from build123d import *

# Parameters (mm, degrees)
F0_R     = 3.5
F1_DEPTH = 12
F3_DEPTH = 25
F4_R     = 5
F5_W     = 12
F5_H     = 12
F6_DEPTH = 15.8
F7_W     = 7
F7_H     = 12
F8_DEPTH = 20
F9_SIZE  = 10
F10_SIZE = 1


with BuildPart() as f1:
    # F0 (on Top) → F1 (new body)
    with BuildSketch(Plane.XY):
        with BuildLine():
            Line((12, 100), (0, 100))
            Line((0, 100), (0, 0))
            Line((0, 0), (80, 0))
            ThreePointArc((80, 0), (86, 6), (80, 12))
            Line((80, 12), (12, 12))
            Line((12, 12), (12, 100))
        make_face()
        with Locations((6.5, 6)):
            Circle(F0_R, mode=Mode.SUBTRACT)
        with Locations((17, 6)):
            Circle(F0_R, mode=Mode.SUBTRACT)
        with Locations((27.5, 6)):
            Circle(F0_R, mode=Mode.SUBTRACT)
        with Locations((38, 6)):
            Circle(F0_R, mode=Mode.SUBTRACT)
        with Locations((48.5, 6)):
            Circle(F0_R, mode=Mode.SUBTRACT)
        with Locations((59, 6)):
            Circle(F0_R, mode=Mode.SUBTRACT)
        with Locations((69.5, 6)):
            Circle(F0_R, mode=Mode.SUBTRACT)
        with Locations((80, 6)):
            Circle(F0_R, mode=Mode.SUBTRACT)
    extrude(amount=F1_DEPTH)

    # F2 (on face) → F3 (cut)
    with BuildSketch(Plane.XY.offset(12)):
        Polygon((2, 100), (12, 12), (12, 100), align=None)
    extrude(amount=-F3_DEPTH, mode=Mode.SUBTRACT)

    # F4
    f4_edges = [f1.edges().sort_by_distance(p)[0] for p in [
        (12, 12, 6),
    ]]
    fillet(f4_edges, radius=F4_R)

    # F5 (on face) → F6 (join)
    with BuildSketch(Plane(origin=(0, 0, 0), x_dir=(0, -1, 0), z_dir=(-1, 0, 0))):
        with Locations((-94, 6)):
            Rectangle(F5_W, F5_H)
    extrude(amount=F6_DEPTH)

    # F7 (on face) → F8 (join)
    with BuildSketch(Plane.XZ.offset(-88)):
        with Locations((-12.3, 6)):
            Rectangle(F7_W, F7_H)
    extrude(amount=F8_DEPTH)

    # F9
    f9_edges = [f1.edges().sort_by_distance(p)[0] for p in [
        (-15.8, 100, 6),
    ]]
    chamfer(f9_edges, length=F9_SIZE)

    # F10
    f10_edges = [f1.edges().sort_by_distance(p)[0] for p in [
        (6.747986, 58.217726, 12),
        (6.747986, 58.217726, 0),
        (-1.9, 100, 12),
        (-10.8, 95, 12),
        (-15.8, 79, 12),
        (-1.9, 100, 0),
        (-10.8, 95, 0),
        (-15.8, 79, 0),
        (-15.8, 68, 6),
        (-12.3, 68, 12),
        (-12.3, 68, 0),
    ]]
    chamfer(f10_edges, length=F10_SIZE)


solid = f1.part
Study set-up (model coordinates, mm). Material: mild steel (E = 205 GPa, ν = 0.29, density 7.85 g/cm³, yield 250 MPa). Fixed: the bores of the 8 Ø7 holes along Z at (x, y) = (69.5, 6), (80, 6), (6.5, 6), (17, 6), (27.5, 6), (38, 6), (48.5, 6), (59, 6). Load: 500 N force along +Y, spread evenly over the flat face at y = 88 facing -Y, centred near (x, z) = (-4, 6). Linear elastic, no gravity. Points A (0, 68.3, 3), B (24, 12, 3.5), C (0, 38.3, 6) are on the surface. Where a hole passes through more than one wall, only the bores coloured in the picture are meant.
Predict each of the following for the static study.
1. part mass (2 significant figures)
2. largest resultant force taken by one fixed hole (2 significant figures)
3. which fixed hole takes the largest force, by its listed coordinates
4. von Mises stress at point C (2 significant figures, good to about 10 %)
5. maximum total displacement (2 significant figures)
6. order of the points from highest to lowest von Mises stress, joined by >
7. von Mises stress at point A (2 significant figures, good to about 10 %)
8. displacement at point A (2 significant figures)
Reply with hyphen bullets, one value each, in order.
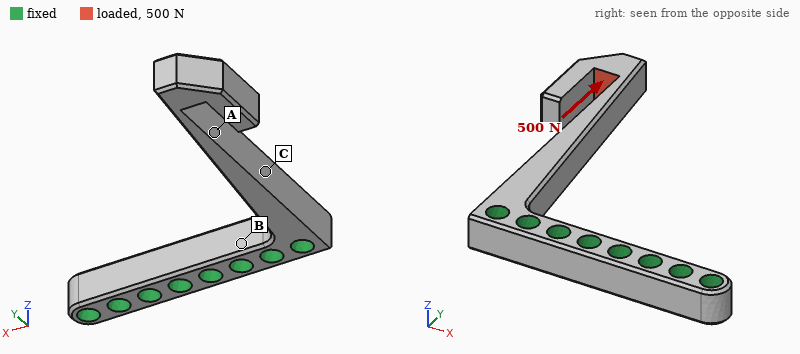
- 150 g
- 780 N
- (6.5, 6)
- 33 MPa
- 0.22 mm
- A > C > B
- 67 MPa
- 0.048 mm
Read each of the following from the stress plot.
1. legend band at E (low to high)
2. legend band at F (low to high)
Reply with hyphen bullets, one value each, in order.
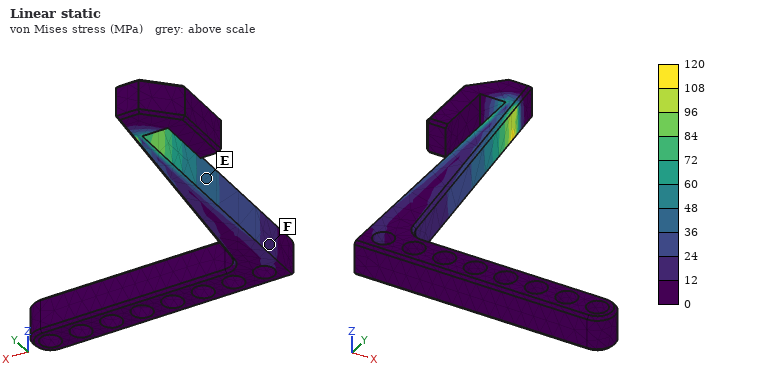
- 36 to 48 MPa
- 12 to 24 MPa
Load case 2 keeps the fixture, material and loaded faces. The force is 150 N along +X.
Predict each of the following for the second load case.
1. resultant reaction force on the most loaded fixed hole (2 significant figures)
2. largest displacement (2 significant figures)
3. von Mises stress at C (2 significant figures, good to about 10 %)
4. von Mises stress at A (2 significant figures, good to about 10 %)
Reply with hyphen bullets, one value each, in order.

- 860 N
- 0.22 mm
- 47 MPa
- 48 MPa
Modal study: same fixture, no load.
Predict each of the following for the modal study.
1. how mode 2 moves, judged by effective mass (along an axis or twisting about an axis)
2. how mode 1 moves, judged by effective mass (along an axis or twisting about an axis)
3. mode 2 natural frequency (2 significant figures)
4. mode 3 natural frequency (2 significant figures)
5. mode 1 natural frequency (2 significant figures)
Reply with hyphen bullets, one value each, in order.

- along Z
- along X
- 990 Hz
- 1900 Hz
- 790 Hz
